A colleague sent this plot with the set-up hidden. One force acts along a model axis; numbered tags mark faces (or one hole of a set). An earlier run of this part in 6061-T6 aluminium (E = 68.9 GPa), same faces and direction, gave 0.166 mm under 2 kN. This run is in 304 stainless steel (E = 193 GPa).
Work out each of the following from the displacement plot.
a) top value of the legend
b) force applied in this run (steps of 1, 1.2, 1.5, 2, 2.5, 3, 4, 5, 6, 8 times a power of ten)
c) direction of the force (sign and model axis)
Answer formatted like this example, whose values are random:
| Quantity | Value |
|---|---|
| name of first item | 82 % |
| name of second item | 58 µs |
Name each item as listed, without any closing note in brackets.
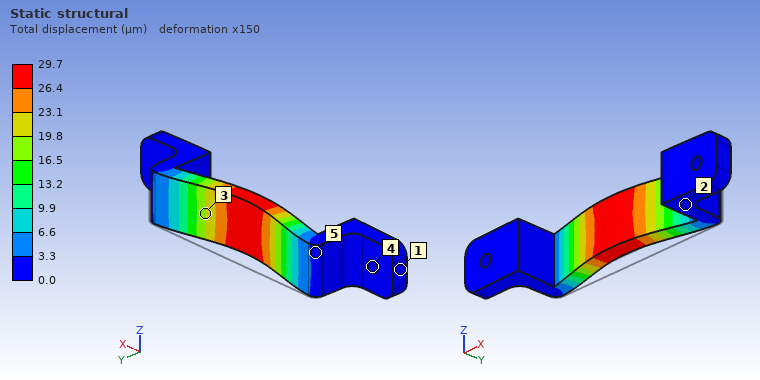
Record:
| Quantity | Value |
|---|---|
| top value of the legend | 29.7 µm |
| force applied in this run | 1 kN |
| direction of the force | -Y |
